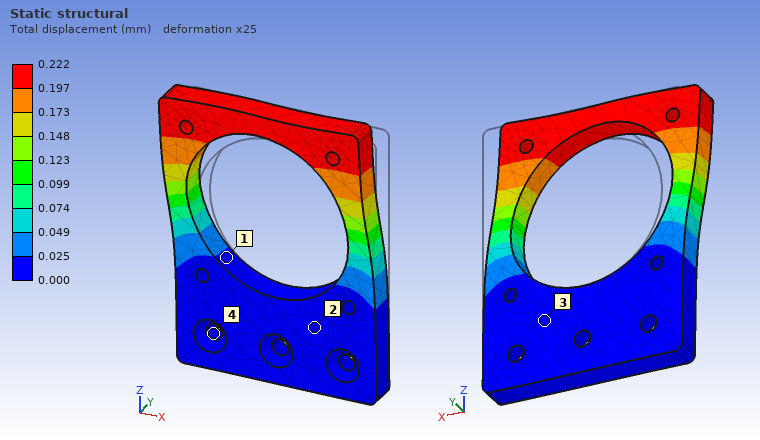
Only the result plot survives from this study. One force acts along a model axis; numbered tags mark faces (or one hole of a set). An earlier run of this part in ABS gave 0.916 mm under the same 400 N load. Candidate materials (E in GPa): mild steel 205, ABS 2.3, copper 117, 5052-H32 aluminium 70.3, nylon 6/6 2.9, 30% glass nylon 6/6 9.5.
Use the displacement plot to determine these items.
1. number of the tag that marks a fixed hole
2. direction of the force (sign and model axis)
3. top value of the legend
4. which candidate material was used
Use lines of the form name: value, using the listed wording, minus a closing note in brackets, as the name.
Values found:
number of the tag that marks a fixed hole: 4
direction of the force: -X
top value of the legend: 0.222 mm
which candidate material was used: 30% glass nylon 6/6
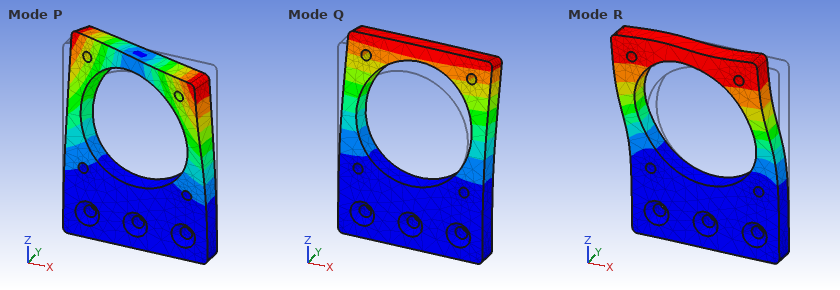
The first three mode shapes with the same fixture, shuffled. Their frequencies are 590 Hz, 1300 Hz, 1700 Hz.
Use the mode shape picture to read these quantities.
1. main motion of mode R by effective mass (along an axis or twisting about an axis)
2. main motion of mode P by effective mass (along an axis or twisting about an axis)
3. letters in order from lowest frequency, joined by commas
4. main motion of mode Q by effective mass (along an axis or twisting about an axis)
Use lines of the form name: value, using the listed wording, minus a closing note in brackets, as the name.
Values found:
main motion of mode R by effective mass: along X
main motion of mode P by effective mass: twisting about Z
letters in order from lowest frequency, joined by commas: Q, P, R
main motion of mode Q by effective mass: along Y
